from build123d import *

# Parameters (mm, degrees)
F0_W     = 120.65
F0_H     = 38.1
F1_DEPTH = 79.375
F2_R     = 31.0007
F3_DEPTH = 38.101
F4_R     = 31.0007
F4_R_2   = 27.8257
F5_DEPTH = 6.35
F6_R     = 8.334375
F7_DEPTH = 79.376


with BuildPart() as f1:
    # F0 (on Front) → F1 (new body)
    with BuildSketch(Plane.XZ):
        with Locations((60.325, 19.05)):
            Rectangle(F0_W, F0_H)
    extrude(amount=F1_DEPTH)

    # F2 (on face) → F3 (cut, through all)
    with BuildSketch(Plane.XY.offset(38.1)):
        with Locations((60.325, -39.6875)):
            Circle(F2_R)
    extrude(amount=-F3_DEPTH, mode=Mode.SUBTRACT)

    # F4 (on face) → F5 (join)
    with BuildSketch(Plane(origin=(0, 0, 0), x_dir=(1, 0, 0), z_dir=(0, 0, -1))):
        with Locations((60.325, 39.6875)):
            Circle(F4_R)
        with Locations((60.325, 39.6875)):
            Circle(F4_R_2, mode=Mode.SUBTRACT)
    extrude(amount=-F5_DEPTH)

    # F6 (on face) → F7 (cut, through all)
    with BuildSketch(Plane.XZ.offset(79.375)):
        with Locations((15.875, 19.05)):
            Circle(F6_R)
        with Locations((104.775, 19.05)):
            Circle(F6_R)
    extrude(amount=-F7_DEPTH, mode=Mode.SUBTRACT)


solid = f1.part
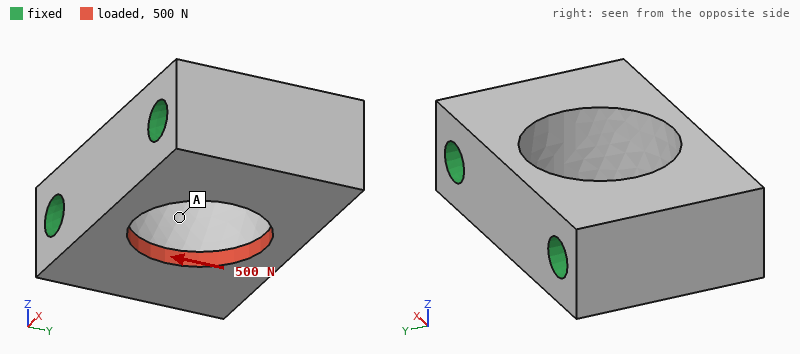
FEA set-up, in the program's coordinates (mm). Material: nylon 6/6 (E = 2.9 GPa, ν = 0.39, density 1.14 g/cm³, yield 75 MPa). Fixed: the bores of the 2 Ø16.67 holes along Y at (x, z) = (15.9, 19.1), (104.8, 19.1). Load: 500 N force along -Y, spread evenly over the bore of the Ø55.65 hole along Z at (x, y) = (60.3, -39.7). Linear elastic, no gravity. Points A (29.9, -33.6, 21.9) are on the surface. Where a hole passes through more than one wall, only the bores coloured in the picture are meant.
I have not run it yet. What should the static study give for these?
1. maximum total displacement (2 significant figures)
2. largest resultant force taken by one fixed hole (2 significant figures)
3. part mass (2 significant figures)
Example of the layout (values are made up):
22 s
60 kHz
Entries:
17 µm
250 N
250 g
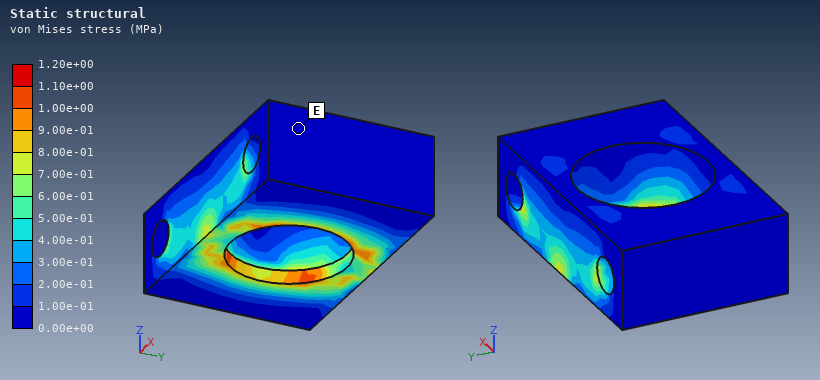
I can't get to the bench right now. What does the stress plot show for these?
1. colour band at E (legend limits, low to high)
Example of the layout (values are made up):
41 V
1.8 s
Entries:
0.00e+00 to 1.00e-01 MPa
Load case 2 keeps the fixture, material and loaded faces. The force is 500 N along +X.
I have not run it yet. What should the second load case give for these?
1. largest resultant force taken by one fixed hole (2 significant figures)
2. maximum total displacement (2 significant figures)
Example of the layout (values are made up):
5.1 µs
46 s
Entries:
250 N
4.4 µm
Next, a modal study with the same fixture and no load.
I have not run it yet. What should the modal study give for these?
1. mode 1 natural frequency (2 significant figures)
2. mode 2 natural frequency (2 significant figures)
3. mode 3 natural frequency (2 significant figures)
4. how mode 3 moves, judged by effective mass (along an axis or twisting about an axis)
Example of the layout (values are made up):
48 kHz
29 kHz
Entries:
5200 Hz
5300 Hz
5700 Hz
along Y
